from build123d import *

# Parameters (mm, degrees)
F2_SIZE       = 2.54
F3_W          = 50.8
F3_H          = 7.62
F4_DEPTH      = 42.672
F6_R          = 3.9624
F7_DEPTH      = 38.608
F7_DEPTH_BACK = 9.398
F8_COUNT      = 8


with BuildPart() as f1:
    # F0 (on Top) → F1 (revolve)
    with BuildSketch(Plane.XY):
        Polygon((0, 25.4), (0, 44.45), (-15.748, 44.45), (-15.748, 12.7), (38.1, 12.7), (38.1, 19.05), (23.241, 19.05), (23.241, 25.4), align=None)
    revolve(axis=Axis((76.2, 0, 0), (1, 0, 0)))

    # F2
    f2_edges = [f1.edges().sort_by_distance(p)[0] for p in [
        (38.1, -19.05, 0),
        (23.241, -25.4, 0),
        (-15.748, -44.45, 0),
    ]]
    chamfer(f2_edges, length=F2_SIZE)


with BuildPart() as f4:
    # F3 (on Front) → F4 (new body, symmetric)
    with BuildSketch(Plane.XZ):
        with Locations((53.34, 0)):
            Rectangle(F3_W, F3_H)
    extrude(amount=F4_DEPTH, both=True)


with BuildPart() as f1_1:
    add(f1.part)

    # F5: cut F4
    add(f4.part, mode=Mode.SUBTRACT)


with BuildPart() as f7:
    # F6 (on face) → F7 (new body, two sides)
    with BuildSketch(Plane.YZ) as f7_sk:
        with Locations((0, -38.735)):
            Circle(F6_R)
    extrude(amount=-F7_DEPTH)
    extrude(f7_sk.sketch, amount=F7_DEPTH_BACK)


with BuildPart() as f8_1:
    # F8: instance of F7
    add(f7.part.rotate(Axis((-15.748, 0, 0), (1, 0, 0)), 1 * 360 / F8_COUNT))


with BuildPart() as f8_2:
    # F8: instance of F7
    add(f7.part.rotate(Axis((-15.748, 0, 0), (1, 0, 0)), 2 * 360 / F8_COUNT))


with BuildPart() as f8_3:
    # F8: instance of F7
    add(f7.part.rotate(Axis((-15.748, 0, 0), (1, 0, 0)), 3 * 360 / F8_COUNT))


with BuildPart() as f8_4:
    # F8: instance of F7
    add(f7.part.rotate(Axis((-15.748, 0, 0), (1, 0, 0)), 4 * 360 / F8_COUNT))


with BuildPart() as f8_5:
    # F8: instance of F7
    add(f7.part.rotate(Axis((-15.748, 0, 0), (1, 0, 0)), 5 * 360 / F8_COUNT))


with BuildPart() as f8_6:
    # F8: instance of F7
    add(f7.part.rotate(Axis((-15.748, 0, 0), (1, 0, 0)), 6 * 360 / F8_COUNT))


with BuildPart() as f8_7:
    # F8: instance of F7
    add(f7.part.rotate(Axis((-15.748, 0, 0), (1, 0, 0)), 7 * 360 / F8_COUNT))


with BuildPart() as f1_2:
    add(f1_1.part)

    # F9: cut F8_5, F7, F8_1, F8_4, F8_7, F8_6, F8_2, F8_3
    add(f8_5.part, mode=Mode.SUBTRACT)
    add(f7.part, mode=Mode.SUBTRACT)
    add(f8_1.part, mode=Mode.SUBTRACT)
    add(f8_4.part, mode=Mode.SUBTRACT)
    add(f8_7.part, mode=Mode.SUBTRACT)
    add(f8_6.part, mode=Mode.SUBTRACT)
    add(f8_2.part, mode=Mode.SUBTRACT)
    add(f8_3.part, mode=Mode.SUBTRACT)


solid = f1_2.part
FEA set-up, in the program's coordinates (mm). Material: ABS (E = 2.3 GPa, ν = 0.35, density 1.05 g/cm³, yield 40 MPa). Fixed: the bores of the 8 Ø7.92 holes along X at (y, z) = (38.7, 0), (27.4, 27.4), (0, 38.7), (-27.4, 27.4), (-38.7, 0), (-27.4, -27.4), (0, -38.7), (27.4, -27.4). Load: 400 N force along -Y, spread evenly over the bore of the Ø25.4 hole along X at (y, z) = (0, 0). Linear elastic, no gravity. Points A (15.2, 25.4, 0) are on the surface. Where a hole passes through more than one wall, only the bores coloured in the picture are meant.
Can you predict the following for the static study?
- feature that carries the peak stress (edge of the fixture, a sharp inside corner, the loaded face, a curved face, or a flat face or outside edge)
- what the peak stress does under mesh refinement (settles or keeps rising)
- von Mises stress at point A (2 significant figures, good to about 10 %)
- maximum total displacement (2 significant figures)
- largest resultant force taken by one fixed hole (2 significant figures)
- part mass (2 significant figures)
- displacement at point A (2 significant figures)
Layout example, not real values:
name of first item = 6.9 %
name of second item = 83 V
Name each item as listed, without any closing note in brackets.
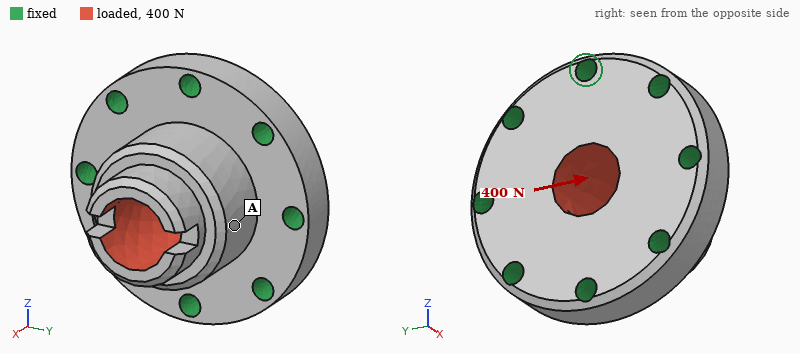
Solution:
feature that carries the peak stress = edge of the fixture
what the peak stress does under mesh refinement = keeps rising
von Mises stress at point A = 0.15 MPa
maximum total displacement = 24 µm
largest resultant force taken by one fixed hole = 99 N
part mass = 130 g
displacement at point A = 11 µm
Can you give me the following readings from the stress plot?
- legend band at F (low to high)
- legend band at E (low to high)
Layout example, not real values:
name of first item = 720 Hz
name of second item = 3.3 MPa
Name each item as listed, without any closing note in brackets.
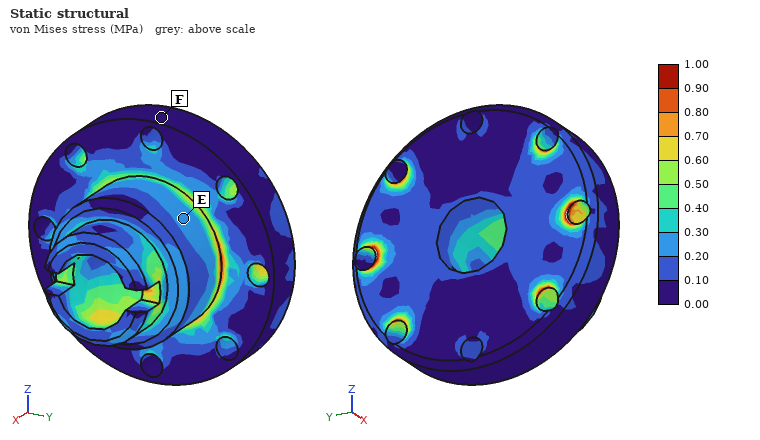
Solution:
legend band at F = 0.00 to 0.10 MPa
legend band at E = 0.20 to 0.30 MPa
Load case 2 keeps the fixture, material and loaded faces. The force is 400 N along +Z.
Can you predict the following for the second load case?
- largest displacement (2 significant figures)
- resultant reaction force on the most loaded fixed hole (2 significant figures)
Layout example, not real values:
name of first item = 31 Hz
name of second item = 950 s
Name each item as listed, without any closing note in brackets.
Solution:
largest displacement = 22 µm
resultant reaction force on the most loaded fixed hole = 99 N
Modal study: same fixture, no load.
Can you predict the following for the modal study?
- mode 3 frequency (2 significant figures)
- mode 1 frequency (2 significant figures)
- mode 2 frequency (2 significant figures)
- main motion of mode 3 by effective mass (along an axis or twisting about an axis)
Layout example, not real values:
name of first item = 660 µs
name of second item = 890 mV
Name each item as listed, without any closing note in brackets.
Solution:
mode 3 frequency = 4900 Hz
mode 1 frequency = 3900 Hz
mode 2 frequency = 3900 Hz
main motion of mode 3 by effective mass = along X
